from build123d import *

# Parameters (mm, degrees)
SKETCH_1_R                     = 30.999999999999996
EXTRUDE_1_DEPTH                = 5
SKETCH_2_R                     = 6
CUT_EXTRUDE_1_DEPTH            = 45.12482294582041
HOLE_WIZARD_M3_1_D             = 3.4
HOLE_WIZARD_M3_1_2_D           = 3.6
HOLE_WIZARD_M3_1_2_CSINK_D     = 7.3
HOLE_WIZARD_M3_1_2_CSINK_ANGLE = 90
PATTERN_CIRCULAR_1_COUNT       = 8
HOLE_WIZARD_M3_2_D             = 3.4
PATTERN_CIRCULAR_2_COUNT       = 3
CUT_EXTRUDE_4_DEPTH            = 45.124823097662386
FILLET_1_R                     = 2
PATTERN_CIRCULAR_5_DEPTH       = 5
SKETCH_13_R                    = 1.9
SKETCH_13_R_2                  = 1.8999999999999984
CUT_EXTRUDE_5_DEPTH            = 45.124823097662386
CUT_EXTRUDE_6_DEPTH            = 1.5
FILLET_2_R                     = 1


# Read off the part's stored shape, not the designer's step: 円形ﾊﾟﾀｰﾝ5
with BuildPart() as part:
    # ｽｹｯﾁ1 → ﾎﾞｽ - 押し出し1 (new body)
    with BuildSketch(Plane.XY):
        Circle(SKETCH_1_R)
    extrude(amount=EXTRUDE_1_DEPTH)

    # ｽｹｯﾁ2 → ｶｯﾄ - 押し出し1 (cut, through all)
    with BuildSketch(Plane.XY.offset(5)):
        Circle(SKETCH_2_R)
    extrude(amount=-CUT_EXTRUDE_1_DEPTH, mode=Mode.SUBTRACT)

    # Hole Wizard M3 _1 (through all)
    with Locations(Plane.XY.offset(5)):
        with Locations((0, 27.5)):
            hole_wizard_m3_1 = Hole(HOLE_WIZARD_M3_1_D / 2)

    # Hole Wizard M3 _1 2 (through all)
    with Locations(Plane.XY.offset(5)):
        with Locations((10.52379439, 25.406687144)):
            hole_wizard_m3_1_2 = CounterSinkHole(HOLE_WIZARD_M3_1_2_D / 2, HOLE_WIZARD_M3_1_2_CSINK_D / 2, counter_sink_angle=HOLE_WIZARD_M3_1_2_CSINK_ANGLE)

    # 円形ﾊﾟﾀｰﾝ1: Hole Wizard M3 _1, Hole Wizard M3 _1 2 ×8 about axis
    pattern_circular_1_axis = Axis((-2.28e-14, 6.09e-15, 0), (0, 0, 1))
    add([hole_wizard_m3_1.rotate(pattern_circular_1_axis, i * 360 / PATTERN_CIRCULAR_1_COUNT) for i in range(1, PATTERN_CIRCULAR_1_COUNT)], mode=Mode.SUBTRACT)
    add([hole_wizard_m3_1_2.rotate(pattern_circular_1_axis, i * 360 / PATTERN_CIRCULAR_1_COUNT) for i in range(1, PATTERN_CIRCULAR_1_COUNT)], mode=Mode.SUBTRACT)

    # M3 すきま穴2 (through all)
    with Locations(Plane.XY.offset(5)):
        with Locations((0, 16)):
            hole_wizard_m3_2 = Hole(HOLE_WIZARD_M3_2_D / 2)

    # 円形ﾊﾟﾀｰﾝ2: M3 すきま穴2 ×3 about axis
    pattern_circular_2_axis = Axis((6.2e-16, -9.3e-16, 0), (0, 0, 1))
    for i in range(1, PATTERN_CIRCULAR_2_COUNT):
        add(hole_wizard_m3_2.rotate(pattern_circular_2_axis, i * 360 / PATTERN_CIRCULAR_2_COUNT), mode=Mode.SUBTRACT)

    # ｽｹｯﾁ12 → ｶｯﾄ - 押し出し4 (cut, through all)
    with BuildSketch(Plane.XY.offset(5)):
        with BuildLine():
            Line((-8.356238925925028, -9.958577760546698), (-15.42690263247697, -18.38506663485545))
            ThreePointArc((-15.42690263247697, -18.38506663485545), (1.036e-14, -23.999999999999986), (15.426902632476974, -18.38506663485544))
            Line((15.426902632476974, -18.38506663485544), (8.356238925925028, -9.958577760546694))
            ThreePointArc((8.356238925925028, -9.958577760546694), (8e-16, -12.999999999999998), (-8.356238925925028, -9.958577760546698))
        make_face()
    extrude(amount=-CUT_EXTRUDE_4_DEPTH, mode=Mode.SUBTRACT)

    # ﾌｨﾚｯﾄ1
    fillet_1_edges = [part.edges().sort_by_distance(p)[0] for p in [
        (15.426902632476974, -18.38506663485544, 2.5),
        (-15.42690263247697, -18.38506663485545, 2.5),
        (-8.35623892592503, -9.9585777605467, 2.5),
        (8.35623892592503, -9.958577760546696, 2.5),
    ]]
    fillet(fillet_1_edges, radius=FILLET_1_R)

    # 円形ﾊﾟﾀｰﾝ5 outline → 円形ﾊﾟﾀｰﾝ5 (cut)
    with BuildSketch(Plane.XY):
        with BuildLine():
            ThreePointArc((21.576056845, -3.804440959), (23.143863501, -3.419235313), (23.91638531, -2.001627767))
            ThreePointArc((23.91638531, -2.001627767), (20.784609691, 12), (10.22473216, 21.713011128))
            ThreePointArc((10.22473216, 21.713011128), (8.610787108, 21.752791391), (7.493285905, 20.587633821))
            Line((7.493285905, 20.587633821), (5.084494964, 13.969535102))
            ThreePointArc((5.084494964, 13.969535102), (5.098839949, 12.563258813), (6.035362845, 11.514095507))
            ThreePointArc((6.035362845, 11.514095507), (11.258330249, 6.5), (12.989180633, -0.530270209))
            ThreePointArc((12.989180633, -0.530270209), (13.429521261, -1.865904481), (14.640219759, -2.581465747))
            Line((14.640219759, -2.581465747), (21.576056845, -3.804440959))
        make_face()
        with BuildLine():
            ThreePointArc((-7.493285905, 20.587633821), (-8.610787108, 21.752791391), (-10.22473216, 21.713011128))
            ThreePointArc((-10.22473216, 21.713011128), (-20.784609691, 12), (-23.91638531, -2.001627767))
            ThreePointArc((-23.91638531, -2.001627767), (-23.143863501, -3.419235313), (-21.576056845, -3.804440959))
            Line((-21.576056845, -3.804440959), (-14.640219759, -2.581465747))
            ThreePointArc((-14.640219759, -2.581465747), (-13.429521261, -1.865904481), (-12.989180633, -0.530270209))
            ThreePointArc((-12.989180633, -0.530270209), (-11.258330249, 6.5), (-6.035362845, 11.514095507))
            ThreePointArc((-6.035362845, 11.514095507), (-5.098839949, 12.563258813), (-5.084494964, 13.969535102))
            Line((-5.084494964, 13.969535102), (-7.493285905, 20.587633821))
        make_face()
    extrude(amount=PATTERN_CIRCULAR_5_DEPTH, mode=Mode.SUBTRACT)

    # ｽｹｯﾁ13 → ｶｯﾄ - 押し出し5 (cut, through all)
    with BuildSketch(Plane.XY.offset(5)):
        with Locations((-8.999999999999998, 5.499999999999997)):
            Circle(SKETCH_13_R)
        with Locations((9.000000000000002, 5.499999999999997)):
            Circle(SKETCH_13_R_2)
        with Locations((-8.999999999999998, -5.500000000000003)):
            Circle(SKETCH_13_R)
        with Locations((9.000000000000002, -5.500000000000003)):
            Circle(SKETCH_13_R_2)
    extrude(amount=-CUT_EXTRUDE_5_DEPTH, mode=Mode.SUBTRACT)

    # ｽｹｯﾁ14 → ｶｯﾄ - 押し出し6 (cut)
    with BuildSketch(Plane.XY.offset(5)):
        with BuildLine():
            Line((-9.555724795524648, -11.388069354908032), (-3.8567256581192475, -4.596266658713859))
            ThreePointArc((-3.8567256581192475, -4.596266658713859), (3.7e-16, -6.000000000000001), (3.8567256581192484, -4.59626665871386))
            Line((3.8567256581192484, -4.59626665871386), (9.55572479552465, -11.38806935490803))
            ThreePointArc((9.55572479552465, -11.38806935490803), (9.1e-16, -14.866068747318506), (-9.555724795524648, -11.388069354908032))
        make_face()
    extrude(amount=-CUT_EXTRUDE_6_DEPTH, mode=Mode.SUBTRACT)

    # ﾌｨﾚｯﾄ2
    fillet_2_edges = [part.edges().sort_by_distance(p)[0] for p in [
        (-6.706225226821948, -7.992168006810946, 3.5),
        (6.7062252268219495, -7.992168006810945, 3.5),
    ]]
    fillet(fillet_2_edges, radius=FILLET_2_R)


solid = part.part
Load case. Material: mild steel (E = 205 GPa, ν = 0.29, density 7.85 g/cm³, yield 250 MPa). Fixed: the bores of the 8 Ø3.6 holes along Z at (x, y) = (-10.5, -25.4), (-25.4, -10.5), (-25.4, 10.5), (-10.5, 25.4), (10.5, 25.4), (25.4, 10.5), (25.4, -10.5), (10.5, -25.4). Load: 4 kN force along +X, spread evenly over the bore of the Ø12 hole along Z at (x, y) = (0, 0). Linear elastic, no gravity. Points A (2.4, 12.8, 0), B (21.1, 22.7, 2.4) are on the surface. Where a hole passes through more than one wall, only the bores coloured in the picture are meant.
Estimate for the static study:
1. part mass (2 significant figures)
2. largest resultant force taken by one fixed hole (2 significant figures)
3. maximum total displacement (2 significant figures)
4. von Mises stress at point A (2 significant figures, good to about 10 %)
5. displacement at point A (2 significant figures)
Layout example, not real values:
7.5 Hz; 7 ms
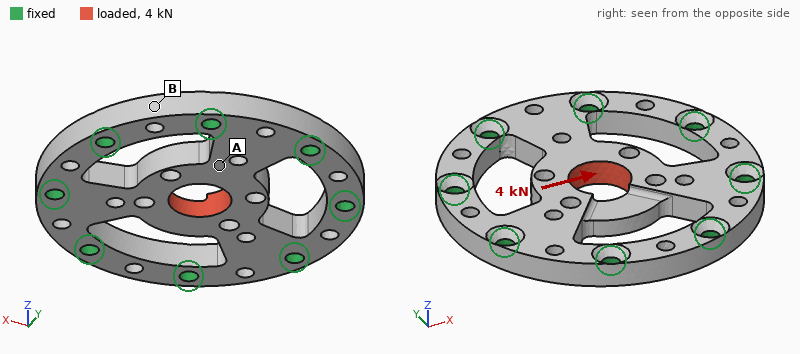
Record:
69 g; 1.5 kN; 9.9 µm; 35 MPa; 5.3 µm
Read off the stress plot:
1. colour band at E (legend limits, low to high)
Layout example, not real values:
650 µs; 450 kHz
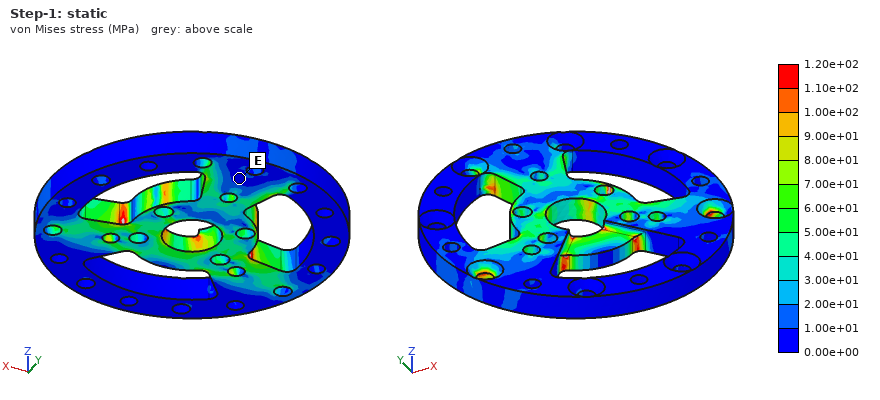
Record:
0.00e+00 to 1.00e+01 MPa
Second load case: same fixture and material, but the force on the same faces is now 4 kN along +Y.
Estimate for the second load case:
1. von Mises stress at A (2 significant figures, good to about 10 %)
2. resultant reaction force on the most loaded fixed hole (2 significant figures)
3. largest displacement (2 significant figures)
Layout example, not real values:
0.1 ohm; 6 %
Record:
34 MPa; 1.1 kN; 12 µm
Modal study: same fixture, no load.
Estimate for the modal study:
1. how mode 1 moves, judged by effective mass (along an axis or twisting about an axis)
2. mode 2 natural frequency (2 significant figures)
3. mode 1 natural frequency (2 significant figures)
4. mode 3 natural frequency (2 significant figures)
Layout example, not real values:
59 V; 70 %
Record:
along Z; 17 kHz; 9100 Hz; 18 kHz
